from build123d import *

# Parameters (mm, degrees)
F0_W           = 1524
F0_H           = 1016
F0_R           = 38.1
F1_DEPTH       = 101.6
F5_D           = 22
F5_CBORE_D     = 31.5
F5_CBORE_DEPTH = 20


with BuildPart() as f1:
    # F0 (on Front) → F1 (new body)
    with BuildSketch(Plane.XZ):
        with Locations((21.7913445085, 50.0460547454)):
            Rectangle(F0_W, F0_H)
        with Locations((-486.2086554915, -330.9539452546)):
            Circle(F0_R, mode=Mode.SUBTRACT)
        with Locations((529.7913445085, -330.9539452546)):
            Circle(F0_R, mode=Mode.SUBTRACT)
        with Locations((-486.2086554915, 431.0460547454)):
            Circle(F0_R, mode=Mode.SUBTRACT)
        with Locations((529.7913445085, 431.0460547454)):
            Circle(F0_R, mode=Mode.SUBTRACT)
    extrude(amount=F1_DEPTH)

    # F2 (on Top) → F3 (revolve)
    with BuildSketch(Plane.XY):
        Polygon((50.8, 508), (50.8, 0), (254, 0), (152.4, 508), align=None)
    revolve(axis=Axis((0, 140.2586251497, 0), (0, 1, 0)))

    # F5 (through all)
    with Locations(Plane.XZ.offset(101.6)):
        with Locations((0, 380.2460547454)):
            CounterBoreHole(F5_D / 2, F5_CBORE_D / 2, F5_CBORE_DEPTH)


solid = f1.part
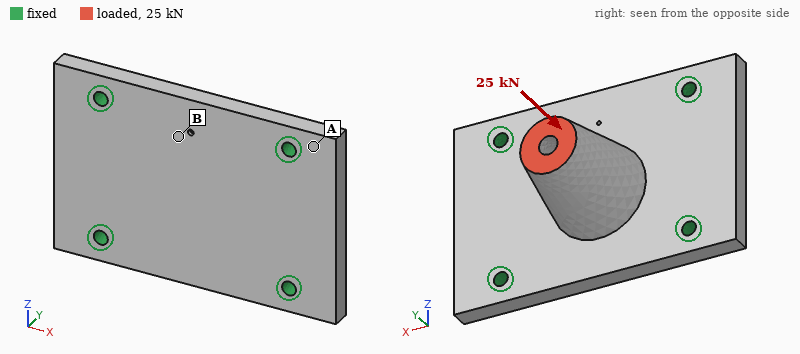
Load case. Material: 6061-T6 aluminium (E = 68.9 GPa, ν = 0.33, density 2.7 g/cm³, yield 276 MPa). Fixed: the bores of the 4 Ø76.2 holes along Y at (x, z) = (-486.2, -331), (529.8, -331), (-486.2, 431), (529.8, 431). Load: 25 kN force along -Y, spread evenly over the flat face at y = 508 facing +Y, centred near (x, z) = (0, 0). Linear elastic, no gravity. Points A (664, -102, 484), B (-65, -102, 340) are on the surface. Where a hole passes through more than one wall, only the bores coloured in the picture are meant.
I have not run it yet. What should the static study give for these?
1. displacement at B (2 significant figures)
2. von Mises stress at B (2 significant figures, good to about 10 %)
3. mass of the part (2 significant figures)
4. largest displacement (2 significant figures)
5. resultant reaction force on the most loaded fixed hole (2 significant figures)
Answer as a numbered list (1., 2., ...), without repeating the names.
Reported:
1. 16 µm
2. 0.66 MPa
3. 590 kg
4. 21 µm
5. 7.7 kN
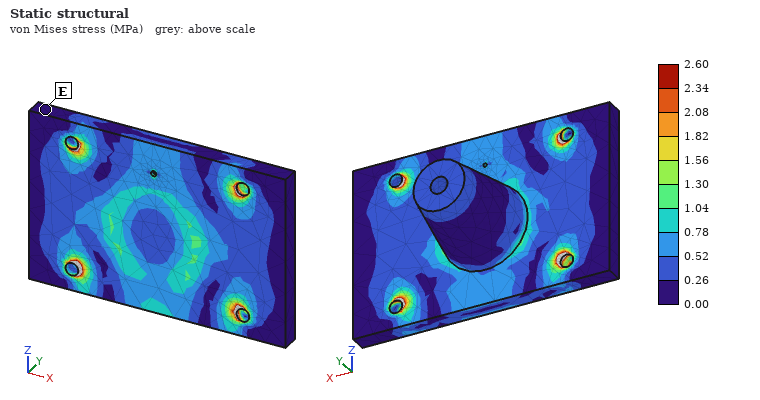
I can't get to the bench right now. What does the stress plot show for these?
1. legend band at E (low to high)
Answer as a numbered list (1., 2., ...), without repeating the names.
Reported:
1. 0.00 to 0.26 MPa
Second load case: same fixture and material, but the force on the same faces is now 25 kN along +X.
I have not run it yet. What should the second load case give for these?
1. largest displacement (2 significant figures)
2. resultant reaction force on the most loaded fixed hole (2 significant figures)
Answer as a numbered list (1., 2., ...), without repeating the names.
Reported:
1. 58 µm
2. 12 kN
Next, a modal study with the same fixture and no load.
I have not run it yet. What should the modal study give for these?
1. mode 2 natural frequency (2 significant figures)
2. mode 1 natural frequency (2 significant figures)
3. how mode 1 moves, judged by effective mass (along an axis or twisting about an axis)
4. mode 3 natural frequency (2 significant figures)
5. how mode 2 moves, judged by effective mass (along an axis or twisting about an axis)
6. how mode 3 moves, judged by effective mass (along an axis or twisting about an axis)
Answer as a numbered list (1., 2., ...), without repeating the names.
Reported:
1. 350 Hz
2. 320 Hz
3. along Y
4. 440 Hz
5. along Z
6. along X
